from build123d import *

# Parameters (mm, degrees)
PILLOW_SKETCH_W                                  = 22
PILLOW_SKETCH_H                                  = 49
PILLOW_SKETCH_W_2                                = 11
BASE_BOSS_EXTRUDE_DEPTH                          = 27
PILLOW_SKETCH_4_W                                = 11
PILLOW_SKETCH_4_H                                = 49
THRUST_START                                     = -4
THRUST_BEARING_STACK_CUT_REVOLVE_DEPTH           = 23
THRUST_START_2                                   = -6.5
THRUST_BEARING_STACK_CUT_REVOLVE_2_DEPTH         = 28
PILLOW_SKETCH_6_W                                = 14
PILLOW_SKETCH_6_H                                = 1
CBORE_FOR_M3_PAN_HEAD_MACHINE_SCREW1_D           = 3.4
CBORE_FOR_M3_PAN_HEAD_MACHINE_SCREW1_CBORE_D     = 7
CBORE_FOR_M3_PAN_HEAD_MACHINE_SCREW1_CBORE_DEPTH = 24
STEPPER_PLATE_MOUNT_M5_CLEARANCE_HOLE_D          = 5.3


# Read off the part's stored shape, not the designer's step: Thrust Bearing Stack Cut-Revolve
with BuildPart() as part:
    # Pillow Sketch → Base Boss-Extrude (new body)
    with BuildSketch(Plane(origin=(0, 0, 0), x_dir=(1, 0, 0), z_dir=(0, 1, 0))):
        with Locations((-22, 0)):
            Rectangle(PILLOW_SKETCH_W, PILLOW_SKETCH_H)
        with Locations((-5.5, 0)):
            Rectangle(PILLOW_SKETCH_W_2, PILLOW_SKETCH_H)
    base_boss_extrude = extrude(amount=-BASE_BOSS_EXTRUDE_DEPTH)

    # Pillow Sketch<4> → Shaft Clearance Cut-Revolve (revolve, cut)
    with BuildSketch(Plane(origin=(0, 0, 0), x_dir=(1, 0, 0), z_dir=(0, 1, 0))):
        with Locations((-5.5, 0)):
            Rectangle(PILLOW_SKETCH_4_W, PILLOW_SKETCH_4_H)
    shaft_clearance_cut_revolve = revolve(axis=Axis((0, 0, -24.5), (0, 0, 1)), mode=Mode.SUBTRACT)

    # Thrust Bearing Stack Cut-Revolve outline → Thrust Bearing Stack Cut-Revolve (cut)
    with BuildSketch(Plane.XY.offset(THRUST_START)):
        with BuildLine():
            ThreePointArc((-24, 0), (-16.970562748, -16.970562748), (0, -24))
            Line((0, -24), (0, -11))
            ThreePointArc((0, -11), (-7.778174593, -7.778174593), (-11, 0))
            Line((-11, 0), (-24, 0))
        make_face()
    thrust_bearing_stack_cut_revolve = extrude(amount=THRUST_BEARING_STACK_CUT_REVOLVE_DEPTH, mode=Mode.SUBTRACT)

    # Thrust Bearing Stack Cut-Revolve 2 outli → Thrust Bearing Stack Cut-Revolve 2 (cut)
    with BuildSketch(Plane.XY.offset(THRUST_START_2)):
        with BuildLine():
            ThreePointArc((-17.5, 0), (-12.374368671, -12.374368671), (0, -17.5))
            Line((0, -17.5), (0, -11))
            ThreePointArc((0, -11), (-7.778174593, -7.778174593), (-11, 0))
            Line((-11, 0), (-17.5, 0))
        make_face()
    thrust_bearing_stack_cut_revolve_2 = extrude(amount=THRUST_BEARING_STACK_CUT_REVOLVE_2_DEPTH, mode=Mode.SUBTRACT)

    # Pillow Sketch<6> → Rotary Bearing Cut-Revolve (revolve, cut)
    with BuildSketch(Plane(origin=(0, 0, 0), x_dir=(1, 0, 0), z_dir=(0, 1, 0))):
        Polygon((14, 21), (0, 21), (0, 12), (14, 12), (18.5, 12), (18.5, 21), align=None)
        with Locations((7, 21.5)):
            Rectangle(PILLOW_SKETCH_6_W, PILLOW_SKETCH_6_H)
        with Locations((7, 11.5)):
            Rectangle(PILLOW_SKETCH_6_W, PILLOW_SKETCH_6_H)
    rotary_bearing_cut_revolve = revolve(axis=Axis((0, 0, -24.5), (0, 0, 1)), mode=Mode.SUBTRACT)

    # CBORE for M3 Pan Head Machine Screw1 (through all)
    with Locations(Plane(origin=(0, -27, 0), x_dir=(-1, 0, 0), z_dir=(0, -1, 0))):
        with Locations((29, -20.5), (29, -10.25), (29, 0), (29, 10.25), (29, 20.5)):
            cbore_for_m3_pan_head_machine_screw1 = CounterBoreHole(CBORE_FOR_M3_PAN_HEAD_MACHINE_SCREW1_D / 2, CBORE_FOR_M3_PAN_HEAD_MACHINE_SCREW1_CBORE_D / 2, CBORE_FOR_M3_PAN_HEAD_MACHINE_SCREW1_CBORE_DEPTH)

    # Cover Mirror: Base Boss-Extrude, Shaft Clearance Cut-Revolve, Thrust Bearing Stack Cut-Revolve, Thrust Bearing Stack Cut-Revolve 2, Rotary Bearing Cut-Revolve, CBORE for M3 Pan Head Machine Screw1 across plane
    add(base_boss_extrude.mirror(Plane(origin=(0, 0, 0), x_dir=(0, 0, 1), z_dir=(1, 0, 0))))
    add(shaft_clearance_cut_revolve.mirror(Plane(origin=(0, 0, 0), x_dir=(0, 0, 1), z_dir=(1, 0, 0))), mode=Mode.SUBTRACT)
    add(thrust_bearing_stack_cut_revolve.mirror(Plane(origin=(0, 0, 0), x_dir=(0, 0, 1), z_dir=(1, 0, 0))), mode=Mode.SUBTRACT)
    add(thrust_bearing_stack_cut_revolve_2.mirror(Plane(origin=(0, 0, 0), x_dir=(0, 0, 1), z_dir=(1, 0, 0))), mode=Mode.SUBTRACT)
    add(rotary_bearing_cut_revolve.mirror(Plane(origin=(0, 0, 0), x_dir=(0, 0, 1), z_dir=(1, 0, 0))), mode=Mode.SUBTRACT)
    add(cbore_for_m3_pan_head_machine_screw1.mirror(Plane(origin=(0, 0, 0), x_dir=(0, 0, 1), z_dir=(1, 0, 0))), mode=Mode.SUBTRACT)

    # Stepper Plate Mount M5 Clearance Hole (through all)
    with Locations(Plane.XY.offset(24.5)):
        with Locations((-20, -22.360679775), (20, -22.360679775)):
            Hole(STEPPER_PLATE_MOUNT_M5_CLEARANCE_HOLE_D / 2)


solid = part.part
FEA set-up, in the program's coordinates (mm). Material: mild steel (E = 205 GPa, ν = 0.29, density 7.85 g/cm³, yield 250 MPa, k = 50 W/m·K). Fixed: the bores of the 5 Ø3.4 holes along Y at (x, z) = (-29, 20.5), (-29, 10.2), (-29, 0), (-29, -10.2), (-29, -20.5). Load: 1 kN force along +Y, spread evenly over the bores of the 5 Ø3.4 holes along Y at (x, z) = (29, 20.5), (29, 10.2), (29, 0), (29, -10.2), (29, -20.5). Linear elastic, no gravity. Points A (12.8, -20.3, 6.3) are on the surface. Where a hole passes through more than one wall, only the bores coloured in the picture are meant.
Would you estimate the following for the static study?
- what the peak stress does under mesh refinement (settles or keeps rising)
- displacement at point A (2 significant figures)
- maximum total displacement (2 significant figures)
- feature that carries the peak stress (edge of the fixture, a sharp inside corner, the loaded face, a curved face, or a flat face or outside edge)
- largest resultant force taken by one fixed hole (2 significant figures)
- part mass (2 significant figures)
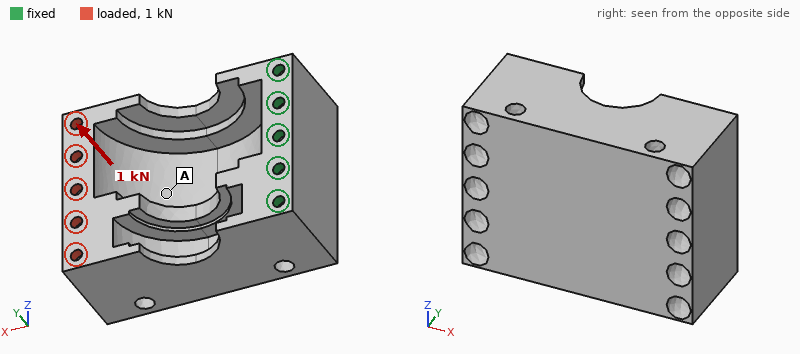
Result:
keeps rising
0.12 mm
0.19 mm
edge of the fixture
620 N
350 g
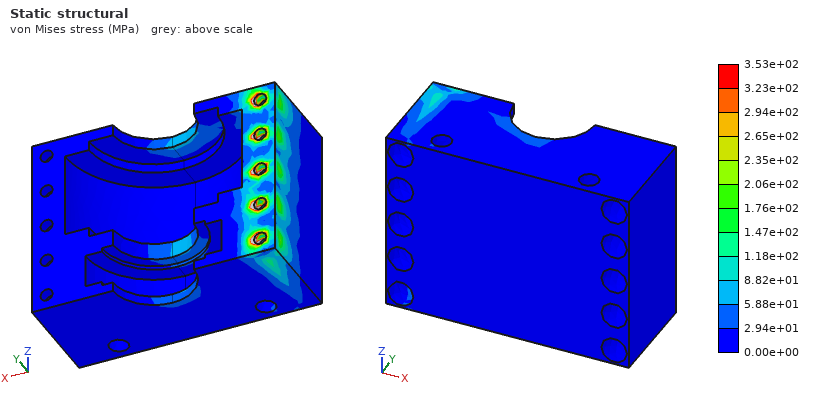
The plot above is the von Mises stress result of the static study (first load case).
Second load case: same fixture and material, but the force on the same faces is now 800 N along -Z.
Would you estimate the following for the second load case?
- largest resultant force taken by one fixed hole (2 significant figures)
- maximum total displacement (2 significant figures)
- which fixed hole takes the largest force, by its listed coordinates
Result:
1.4 kN
48 µm
(-29, -20.5)
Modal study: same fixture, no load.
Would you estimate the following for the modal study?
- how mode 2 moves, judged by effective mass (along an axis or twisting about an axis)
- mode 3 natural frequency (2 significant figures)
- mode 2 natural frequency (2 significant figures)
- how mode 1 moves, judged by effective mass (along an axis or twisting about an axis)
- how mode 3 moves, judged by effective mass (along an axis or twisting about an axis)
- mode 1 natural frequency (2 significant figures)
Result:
along Z
5500 Hz
2300 Hz
along Y
along X
1000 Hz
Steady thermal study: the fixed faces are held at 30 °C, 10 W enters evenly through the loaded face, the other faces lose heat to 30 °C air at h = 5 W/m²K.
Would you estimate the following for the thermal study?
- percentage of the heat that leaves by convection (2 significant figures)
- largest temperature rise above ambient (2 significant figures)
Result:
17 %
34 K
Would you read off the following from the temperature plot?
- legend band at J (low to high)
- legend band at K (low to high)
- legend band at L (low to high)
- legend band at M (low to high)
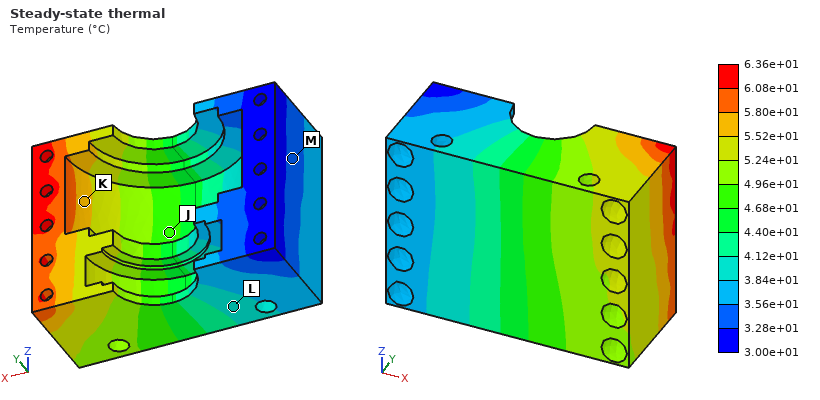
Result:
4.68e+01 to 4.96e+01 °C
5.52e+01 to 5.80e+01 °C
3.84e+01 to 4.12e+01 °C
3.28e+01 to 3.56e+01 °C
